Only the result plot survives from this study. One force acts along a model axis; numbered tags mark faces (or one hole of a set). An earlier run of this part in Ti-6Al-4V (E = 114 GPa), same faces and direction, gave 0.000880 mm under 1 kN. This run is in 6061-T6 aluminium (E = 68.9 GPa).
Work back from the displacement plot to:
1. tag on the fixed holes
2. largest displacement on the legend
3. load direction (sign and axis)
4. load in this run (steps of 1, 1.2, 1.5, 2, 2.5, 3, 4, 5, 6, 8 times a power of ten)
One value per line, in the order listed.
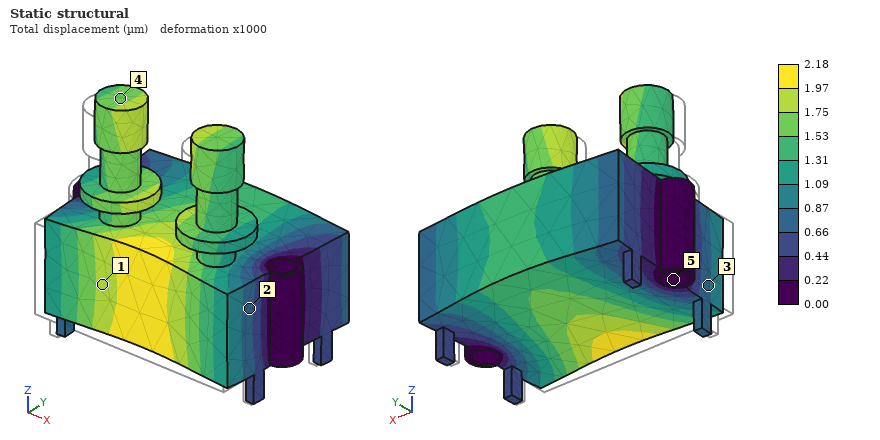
5
2.18 µm
+Y
1.5 kN
